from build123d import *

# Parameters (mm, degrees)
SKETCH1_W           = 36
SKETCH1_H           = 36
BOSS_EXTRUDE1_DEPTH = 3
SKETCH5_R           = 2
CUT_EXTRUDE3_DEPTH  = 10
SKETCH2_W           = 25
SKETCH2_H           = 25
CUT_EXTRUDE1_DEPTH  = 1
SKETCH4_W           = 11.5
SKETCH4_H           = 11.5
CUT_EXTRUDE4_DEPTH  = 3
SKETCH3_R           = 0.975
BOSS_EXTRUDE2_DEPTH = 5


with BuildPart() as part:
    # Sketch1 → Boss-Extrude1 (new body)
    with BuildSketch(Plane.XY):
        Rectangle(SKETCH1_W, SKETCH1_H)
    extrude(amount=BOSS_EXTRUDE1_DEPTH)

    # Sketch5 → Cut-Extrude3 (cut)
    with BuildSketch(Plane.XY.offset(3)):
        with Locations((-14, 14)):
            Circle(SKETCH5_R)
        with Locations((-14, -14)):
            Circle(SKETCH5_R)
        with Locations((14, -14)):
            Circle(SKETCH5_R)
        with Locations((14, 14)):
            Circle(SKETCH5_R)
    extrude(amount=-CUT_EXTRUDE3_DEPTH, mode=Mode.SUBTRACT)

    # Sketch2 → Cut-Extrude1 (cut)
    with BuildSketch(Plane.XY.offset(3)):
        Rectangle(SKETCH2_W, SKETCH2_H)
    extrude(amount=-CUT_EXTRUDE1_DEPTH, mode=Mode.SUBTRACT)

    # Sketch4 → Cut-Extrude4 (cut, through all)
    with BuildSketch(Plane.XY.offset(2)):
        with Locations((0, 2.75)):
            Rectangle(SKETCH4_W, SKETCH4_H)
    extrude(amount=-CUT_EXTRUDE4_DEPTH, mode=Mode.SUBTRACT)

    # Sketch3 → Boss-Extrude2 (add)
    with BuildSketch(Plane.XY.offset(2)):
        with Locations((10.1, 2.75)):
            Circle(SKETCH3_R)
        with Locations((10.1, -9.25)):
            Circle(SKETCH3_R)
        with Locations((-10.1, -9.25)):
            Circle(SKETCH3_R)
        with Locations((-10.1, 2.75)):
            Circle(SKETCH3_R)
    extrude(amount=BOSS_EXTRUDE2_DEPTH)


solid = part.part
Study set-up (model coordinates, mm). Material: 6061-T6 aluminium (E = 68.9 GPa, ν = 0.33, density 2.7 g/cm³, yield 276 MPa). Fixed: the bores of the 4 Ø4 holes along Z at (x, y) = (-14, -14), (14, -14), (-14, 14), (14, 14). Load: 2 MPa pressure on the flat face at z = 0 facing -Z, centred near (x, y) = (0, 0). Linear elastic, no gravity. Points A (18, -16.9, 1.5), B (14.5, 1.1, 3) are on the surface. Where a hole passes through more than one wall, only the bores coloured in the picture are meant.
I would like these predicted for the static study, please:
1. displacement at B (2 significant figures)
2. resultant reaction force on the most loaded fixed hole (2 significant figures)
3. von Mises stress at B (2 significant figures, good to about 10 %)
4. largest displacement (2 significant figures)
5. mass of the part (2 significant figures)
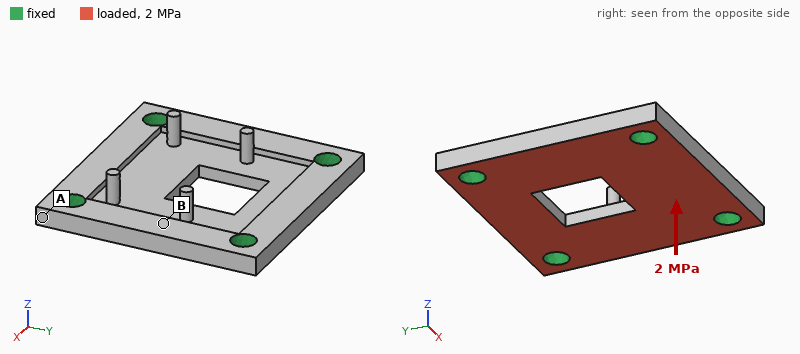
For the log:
25 µm
580 N
60 MPa
79 µm
7.9 g
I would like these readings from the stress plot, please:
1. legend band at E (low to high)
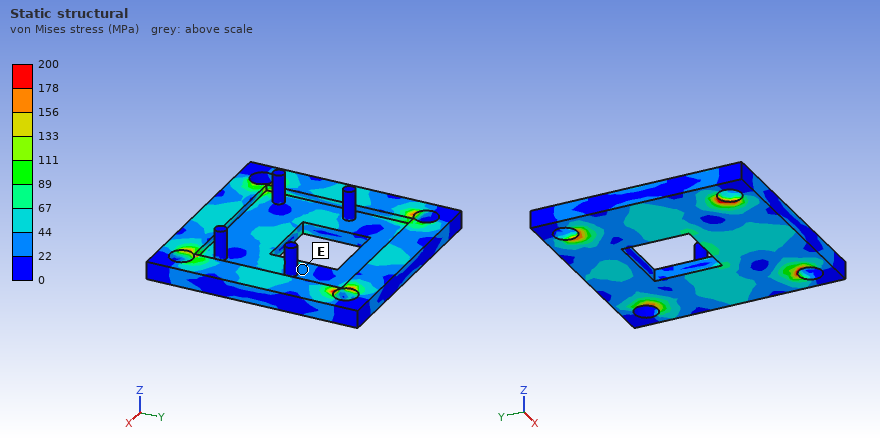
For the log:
22 to 44 MPa
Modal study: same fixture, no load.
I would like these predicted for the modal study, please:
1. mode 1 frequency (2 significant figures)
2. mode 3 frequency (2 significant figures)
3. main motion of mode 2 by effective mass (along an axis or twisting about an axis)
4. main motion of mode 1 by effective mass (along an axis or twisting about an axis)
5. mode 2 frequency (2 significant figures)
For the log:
15 kHz
21 kHz
twisting about Y
along Z
20 kHz
